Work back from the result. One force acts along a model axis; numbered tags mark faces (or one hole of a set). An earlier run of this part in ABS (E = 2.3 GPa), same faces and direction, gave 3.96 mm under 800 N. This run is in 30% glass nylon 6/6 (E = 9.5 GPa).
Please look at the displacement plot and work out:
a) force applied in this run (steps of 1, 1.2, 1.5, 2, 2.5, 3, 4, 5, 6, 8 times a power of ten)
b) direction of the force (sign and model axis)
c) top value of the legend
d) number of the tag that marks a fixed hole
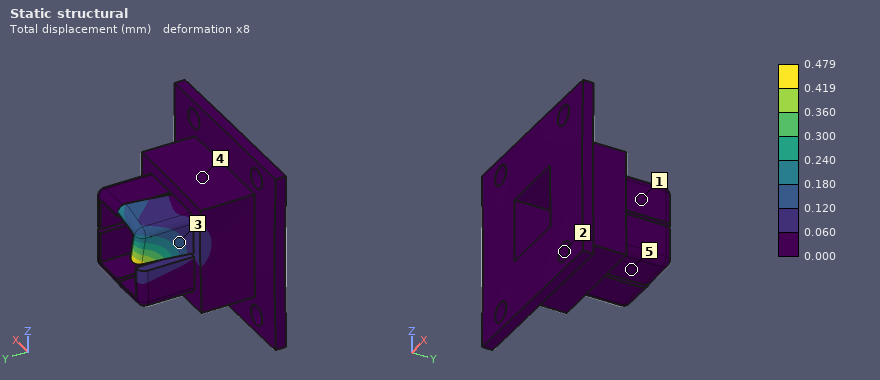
400 N
+X
0.479 mm
2
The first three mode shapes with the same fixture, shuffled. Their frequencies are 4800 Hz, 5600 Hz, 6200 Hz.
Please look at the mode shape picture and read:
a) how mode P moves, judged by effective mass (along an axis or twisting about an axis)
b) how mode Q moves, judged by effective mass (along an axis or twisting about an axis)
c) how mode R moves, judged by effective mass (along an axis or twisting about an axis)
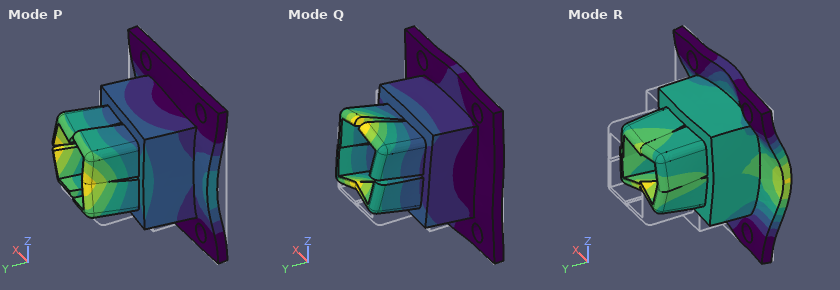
along X
along Z
along Y
